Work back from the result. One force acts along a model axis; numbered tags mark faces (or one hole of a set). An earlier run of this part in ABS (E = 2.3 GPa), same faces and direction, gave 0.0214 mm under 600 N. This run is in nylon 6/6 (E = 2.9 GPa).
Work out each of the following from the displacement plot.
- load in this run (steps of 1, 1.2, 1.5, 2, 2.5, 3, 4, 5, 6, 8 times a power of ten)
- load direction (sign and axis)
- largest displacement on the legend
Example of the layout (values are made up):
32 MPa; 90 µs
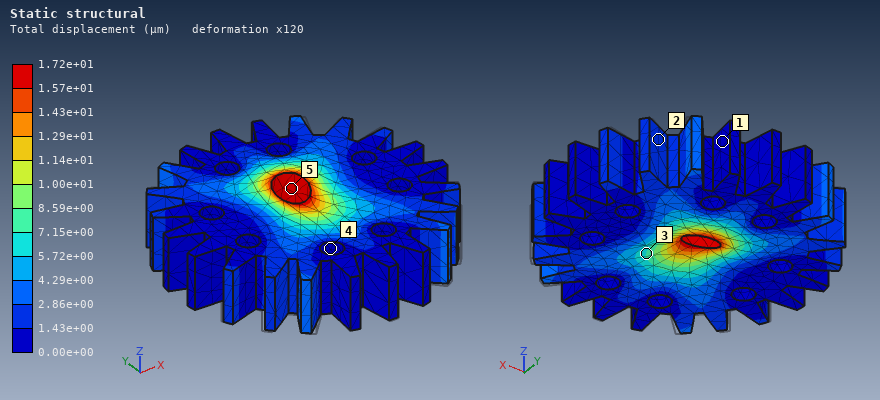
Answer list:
600 N; +Y; 1.72e+01 µm
